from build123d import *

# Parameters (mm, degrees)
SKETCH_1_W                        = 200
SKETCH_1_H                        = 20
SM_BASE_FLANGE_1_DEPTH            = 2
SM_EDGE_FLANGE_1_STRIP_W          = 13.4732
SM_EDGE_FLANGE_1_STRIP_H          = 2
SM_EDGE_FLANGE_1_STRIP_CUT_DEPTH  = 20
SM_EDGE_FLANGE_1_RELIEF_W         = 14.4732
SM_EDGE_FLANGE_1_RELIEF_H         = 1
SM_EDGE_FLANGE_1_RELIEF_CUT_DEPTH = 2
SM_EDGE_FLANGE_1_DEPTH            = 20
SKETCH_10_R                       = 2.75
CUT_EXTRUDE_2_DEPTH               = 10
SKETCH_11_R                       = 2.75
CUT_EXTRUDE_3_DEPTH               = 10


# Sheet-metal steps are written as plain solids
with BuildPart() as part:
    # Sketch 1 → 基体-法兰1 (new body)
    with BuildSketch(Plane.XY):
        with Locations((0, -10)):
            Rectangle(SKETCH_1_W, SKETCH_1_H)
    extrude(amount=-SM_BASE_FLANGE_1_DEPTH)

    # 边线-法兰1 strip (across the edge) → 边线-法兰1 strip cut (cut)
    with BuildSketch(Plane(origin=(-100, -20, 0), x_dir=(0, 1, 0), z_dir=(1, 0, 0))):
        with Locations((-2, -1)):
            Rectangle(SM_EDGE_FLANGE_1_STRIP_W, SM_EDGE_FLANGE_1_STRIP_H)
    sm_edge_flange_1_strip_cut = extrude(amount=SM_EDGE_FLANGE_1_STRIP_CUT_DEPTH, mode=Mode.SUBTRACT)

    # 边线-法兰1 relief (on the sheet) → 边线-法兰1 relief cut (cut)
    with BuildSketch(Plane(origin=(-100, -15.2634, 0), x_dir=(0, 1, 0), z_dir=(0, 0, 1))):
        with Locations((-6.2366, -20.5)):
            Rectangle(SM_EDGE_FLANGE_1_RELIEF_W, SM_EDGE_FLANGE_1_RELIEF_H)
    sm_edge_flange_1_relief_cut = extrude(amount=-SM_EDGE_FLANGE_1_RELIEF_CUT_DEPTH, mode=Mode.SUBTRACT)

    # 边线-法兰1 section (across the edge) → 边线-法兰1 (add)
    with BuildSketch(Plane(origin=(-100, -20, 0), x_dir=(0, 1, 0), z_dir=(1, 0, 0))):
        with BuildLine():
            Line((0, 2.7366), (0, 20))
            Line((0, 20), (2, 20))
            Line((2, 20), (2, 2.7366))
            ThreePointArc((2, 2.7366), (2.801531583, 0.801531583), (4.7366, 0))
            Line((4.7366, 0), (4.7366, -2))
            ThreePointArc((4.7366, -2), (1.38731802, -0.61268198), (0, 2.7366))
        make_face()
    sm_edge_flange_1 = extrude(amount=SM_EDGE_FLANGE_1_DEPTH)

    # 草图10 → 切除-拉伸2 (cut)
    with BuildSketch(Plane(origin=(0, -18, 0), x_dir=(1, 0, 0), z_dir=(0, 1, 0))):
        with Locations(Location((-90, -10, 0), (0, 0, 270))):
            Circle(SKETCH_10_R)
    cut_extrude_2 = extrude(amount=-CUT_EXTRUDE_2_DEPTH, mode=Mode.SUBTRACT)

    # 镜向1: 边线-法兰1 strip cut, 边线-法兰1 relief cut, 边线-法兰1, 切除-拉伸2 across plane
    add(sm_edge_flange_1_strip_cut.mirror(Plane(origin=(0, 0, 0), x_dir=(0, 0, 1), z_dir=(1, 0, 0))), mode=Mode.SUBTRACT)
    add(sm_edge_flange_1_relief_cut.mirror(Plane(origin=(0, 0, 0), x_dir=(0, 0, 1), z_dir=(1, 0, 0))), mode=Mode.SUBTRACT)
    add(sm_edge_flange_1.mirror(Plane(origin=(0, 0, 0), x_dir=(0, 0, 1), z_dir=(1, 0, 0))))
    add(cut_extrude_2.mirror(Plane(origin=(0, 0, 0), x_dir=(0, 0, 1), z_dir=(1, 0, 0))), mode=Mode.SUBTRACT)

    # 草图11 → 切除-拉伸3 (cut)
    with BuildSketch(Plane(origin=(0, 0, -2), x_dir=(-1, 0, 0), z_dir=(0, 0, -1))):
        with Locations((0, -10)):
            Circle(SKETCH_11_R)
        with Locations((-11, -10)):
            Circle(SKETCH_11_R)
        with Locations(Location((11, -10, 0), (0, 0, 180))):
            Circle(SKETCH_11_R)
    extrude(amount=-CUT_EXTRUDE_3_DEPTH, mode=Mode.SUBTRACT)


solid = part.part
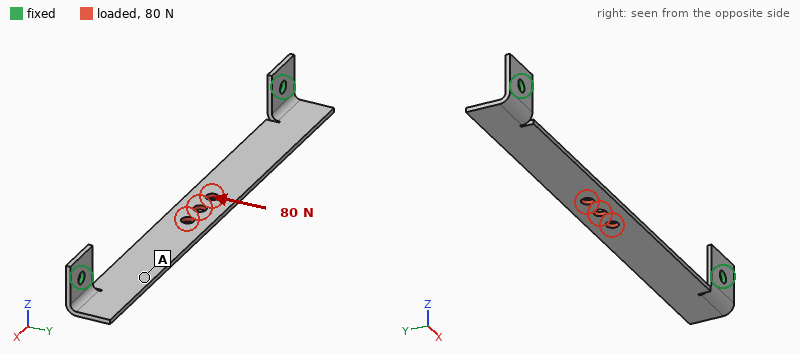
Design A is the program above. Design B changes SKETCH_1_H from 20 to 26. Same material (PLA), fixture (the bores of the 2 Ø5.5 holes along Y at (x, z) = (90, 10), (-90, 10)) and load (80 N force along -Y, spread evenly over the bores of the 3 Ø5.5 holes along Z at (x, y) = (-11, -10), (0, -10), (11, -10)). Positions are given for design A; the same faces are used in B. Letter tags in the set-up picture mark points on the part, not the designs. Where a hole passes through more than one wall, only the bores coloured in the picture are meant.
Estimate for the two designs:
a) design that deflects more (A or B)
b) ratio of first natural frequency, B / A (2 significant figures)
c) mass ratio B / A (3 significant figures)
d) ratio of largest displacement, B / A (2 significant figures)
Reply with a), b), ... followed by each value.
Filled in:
a) A
b) 0.96
c) 1.23
d) 0.76
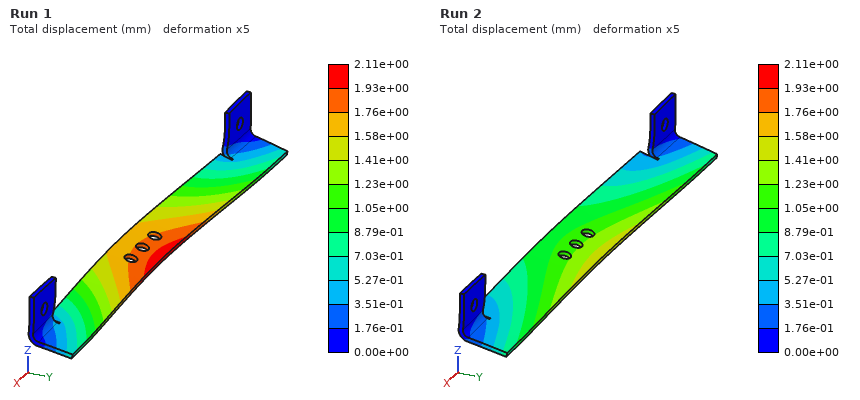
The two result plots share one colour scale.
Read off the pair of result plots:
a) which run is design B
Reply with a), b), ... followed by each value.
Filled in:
a) Run 2
